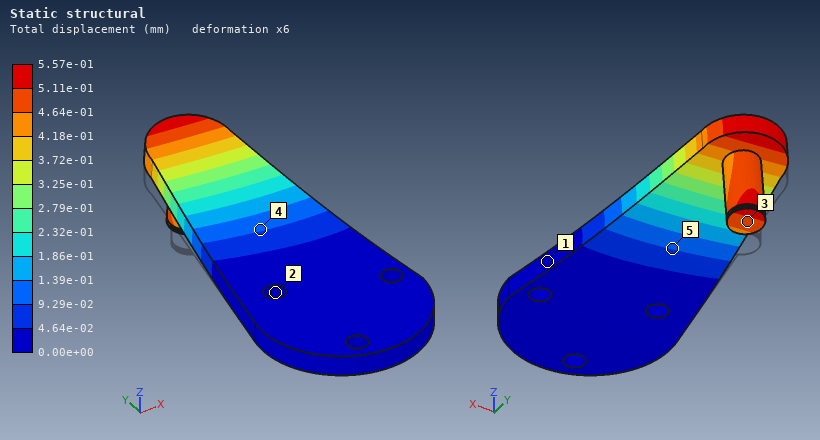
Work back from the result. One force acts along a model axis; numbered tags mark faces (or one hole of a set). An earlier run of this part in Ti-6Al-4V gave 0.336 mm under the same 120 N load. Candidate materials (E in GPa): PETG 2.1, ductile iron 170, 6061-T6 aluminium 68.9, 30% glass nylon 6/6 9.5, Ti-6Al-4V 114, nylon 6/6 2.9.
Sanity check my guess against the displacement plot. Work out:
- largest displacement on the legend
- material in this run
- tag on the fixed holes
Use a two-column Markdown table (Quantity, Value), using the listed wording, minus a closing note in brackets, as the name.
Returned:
| Quantity | Value |
|---|---|
| largest displacement on the legend | 5.57e-01 mm |
| material in this run | 6061-T6 aluminium |
| tag on the fixed holes | 2 |
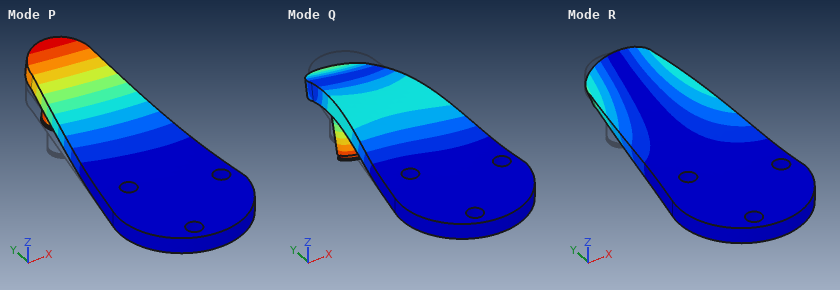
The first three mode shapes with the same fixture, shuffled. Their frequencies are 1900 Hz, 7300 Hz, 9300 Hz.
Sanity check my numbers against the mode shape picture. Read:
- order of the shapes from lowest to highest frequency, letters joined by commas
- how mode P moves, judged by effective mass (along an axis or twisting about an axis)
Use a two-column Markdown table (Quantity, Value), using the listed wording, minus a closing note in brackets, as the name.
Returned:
| Quantity | Value |
|---|---|
| order of the shapes from lowest to highest frequency, letters joined by commas | P, R, Q |
| how mode P moves, judged by effective mass | along Z |
